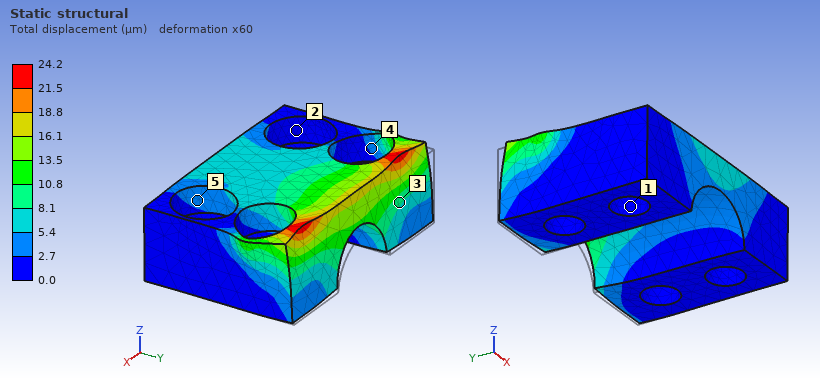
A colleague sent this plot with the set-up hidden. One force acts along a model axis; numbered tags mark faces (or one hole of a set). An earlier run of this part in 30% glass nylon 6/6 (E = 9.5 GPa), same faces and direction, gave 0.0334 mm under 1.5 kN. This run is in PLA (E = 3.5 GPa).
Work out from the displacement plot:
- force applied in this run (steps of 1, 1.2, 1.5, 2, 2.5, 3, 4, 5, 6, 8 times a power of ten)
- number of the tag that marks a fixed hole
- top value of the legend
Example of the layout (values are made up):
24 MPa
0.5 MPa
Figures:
400 N
1
24.2 µm
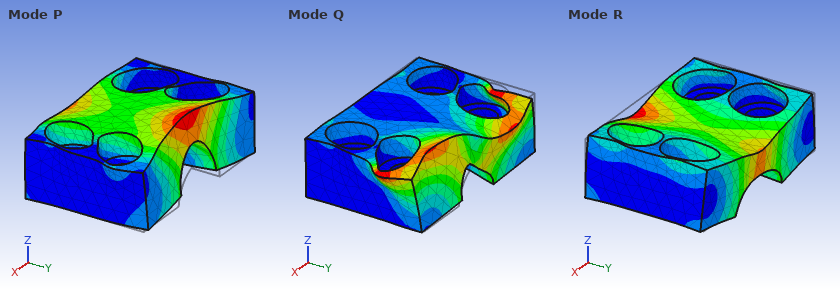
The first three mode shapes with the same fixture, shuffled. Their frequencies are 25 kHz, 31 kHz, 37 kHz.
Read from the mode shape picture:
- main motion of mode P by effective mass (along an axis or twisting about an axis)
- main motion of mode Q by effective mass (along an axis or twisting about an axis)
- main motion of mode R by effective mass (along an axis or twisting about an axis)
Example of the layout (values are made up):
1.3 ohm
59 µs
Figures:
along Y
along X
along Z
